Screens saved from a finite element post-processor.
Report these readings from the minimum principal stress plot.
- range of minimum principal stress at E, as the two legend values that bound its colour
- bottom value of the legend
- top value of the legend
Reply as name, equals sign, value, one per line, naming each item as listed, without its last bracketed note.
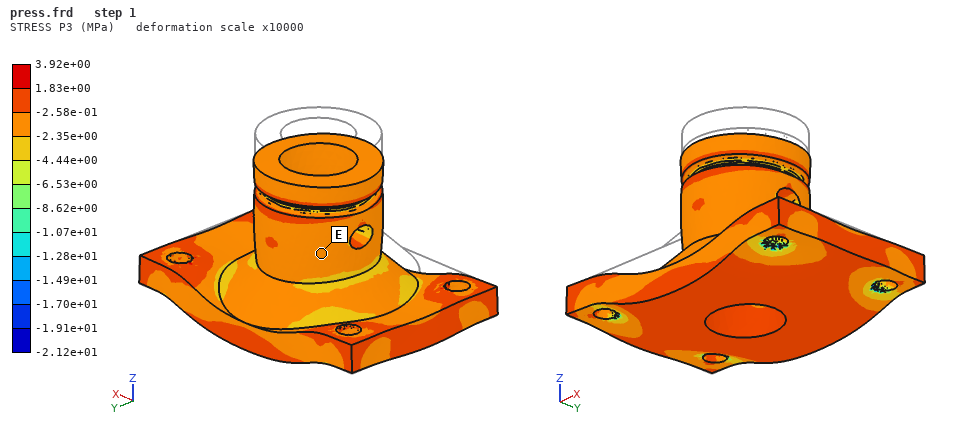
range of minimum principal stress at E, as the two legend values that bound its colour = -2.35e+00 to -2.58e-01 MPa
bottom value of the legend = -2.12e+01 MPa
top value of the legend = 3.92e+00 MPa
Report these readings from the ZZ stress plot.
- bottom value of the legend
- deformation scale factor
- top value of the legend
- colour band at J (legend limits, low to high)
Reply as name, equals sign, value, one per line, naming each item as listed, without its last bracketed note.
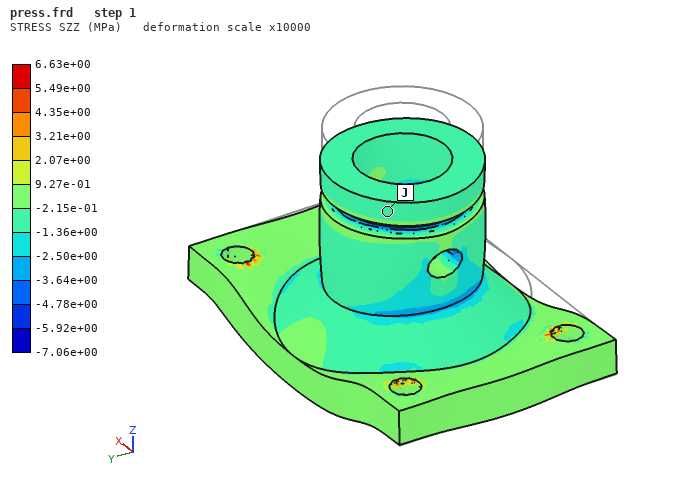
bottom value of the legend = -7.06e+00 MPa
deformation scale factor = 10000
top value of the legend = 6.63e+00 MPa
colour band at J = -1.36e+00 to -2.15e-01 MPa
